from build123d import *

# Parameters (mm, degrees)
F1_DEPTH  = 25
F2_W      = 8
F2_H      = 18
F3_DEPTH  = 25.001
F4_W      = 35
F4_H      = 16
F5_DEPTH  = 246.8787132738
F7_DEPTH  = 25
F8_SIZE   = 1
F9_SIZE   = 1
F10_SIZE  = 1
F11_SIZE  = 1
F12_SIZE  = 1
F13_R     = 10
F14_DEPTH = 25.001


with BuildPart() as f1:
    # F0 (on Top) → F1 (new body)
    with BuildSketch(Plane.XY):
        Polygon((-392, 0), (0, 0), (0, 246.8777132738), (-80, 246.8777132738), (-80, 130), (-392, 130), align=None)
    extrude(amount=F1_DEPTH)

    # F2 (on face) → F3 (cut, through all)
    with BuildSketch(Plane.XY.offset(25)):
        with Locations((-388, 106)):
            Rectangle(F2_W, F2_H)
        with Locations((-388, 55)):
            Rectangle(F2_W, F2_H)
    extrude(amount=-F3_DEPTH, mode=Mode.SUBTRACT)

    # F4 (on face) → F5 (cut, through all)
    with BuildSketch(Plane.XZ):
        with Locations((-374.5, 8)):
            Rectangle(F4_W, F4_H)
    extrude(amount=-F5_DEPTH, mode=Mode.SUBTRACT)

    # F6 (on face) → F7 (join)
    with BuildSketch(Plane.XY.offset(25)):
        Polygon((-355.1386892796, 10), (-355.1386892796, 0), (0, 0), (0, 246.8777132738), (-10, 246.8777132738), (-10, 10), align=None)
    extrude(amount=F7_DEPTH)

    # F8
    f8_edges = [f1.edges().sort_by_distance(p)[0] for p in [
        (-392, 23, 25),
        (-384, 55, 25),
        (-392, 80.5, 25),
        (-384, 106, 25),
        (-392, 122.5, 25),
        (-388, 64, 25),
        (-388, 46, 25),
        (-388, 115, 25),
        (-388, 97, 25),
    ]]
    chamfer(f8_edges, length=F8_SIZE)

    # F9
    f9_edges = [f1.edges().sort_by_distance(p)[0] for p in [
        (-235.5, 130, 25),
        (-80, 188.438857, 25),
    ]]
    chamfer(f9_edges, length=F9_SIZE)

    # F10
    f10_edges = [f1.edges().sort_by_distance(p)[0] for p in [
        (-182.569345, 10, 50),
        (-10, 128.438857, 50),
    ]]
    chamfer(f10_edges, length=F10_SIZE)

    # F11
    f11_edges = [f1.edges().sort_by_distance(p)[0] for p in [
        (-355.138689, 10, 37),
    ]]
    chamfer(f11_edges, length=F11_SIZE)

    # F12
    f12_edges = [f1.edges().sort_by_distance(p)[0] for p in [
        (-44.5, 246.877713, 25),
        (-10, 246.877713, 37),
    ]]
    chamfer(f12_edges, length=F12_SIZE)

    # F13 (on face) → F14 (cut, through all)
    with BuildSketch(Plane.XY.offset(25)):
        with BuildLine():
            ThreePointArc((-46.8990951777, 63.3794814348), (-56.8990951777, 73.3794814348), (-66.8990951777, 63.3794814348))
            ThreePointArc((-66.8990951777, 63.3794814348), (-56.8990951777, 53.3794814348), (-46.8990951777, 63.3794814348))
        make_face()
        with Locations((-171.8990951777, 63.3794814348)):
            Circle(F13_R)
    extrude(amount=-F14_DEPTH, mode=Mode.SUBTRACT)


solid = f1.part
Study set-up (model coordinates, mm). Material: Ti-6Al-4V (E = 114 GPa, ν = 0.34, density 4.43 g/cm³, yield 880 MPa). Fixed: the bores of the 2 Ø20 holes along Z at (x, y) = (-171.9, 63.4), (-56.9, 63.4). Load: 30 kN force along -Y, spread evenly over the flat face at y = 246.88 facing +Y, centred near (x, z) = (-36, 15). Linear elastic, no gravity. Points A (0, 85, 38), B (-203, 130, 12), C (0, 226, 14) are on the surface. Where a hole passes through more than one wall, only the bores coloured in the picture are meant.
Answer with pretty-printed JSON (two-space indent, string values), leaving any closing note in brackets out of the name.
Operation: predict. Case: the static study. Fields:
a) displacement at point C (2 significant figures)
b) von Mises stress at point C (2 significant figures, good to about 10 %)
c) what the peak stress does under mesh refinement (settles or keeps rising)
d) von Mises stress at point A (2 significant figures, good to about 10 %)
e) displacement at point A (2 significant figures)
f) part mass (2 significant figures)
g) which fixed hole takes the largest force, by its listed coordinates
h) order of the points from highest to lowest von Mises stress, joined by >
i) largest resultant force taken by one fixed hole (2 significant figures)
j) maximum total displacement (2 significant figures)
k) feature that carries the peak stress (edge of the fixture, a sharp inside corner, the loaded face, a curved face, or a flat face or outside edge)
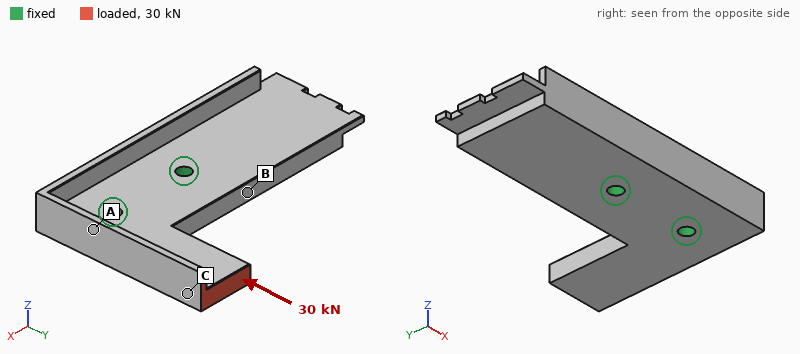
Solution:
{
  "displacement at point C": "46 µm",
  "von Mises stress at point C": "14 MPa",
  "what the peak stress does under mesh refinement": "keeps rising",
  "von Mises stress at point A": "8.2 MPa",
  "displacement at point A": "20 µm",
  "part mass": "6.9 kg",
  "which fixed hole takes the largest force, by its listed coordinates": "(-56.9, 63.4)",
  "order of the points from highest to lowest von Mises stress, joined by >": "C > A > B",
  "largest resultant force taken by one fixed hole": "34 kN",
  "maximum total displacement": "51 µm",
  "feature that carries the peak stress": "edge of the fixture"
}
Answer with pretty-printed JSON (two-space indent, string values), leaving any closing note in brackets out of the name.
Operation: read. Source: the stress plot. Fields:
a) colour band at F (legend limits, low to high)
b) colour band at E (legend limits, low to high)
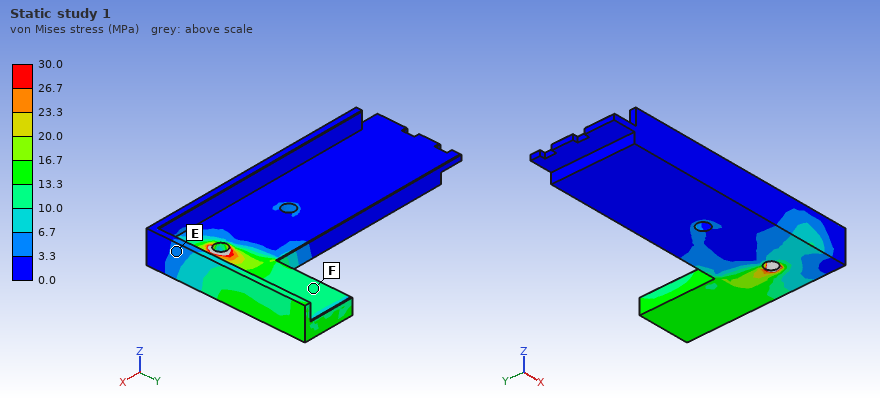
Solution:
{
  "colour band at F": "10.0 to 13.3 MPa",
  "colour band at E": "3.3 to 6.7 MPa"
}
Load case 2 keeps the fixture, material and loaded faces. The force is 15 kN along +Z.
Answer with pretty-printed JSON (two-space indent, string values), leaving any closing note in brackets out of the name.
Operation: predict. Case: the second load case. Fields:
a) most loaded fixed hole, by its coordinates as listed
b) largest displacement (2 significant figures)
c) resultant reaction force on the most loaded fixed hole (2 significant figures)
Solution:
{
  "most loaded fixed hole, by its coordinates as listed": "(-56.9, 63.4)",
  "largest displacement": "1.5 mm",
  "resultant reaction force on the most loaded fixed hole": "16 kN"
}
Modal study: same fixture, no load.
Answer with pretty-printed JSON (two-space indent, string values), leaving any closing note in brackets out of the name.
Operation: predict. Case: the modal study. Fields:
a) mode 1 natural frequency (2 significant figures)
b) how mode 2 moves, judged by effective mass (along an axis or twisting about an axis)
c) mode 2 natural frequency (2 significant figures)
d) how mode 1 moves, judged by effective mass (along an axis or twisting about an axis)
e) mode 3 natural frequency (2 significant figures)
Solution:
{
  "mode 1 natural frequency": "580 Hz",
  "how mode 2 moves, judged by effective mass": "along Z",
  "mode 2 natural frequency": "730 Hz",
  "how mode 1 moves, judged by effective mass": "along Z",
  "mode 3 natural frequency": "1300 Hz"
}
